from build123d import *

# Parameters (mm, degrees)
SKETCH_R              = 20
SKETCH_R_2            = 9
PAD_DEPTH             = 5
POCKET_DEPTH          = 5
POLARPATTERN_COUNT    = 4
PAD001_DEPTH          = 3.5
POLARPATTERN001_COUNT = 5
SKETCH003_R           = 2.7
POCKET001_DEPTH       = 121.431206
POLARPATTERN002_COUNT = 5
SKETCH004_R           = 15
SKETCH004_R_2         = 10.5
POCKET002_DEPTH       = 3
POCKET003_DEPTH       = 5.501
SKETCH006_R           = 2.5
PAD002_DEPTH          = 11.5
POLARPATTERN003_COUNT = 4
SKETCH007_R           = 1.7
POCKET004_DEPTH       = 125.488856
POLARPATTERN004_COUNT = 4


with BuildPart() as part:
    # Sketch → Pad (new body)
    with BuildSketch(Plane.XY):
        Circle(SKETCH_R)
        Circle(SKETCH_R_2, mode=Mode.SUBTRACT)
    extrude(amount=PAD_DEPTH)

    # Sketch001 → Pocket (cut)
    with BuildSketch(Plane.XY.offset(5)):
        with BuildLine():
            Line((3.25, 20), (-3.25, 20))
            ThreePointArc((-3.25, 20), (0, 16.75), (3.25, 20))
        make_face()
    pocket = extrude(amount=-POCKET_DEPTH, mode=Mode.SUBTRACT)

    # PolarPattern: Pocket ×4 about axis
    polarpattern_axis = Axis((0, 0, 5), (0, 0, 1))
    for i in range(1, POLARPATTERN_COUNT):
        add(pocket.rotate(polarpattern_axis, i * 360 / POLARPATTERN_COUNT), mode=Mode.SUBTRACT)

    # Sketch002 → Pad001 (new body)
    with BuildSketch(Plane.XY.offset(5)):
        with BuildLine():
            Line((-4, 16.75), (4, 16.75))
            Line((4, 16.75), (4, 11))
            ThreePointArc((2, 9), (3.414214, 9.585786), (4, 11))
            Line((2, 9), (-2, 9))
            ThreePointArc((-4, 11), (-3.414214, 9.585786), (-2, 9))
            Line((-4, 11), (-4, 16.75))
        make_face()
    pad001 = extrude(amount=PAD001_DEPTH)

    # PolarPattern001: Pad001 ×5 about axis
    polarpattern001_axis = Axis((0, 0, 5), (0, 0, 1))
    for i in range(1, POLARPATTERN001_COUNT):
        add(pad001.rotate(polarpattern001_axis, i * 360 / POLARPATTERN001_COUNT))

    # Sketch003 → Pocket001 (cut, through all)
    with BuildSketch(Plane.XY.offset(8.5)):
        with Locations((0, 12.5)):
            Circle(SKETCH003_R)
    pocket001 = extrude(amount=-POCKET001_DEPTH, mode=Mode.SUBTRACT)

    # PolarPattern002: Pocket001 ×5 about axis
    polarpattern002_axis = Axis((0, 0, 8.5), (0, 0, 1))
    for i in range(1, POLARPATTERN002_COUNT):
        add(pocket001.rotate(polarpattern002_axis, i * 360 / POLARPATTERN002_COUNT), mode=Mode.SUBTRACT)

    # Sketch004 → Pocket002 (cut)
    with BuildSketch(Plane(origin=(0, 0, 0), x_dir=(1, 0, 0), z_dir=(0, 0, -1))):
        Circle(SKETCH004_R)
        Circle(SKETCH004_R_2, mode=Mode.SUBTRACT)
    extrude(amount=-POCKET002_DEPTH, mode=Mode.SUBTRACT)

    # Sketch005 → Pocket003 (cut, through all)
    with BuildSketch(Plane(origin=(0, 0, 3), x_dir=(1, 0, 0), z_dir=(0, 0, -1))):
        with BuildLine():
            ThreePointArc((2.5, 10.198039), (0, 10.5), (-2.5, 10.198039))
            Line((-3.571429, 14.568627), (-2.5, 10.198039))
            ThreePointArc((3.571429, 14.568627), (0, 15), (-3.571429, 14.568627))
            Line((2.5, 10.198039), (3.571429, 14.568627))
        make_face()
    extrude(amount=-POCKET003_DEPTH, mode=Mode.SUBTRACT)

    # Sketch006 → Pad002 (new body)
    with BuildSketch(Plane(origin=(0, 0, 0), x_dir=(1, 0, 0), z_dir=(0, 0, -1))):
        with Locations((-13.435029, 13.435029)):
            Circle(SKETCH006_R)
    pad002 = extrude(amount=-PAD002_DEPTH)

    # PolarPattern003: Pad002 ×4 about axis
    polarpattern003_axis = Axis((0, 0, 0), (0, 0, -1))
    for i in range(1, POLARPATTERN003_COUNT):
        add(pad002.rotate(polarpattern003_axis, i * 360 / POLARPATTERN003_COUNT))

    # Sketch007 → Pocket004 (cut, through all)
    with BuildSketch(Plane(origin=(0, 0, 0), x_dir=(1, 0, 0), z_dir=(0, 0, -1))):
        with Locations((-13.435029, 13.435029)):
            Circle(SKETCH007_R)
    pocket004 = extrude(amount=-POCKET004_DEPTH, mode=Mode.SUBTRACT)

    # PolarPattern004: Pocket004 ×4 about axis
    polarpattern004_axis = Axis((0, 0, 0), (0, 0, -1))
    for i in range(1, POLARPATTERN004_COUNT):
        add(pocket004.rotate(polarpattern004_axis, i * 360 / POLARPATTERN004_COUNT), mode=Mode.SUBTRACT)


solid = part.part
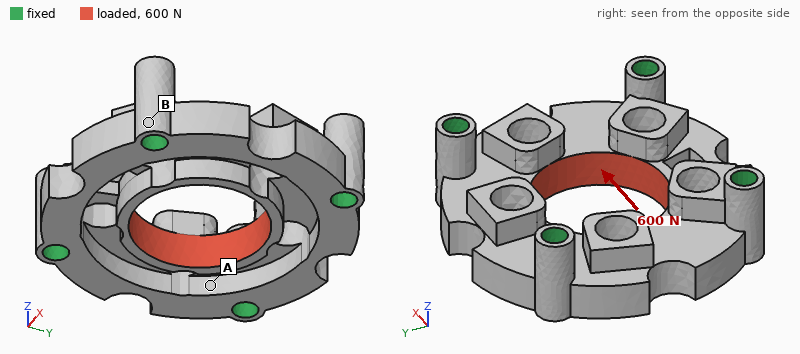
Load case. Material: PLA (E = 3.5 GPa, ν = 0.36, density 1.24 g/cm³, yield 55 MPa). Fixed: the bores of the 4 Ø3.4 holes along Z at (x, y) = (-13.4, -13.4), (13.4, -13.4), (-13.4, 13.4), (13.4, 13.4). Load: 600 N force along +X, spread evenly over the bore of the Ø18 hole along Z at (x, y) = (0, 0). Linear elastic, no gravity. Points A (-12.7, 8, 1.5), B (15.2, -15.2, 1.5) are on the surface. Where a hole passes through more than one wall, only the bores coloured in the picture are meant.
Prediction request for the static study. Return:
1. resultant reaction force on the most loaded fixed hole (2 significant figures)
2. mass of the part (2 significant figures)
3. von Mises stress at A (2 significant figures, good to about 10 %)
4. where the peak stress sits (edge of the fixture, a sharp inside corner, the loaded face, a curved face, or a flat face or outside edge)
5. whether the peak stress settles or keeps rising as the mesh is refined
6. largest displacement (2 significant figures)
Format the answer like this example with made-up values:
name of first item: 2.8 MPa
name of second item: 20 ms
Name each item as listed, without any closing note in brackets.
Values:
resultant reaction force on the most loaded fixed hole: 160 N
mass of the part: 5.1 g
von Mises stress at A: 7.0 MPa
where the peak stress sits: a sharp inside corner
whether the peak stress settles or keeps rising as the mesh is refined: keeps rising
largest displacement: 0.13 mm
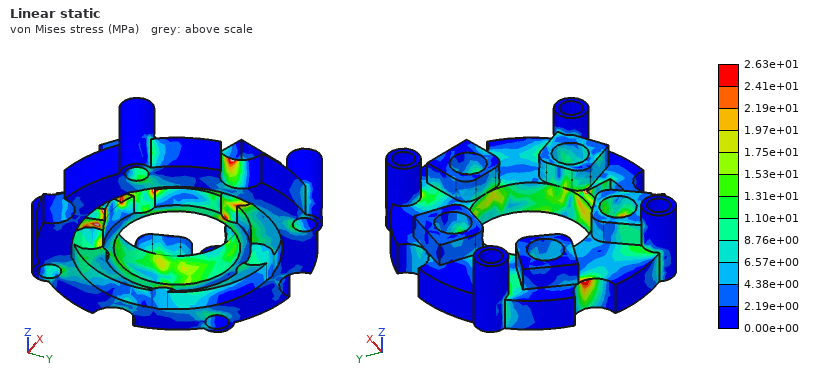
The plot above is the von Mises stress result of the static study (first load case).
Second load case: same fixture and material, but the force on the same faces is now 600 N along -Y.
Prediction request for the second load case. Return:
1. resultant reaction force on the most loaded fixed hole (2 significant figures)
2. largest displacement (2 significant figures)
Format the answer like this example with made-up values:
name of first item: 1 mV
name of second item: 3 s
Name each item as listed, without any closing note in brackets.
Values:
resultant reaction force on the most loaded fixed hole: 170 N
largest displacement: 0.12 mm
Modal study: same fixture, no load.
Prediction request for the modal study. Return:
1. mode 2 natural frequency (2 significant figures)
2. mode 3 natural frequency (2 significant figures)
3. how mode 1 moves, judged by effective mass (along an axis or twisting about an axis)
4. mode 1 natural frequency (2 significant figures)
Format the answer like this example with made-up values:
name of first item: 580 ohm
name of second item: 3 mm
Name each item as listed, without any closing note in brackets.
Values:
mode 2 natural frequency: 9300 Hz
mode 3 natural frequency: 9800 Hz
how mode 1 moves, judged by effective mass: along Z
mode 1 natural frequency: 8700 Hz
